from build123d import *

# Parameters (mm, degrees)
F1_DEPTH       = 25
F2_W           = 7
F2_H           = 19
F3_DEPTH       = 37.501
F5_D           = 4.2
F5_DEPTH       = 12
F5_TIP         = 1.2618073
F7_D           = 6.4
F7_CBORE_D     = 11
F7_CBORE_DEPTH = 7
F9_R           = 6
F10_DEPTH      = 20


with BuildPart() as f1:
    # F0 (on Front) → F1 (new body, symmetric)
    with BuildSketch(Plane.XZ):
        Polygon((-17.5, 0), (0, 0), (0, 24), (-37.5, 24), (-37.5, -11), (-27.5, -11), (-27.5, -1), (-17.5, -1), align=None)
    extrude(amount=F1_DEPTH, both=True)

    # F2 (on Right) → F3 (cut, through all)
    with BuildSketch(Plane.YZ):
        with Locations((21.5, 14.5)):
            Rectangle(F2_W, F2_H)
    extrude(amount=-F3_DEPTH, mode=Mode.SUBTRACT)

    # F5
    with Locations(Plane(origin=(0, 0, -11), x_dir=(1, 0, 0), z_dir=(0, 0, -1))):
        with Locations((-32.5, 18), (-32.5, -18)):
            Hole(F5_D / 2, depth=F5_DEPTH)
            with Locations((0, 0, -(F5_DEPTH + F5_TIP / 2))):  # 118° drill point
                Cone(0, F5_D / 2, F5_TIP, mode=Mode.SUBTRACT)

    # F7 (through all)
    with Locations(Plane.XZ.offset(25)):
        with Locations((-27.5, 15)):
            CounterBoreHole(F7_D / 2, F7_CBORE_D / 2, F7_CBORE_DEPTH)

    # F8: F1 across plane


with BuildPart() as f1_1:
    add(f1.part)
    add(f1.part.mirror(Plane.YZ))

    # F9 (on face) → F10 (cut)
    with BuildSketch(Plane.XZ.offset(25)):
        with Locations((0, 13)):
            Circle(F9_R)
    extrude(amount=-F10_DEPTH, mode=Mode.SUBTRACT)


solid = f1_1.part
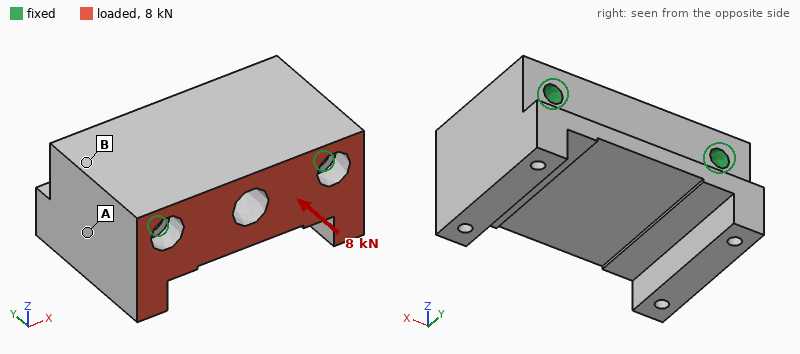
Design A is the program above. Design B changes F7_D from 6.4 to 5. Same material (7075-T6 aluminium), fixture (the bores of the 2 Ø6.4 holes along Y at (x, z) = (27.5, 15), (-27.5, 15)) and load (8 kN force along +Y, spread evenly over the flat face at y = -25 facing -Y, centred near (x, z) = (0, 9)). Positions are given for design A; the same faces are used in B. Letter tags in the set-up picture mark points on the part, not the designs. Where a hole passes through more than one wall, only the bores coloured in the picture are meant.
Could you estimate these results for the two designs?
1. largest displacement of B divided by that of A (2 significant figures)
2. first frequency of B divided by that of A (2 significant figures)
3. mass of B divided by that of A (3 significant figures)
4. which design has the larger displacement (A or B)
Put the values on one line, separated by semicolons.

1.1; 0.92; 1.01; B
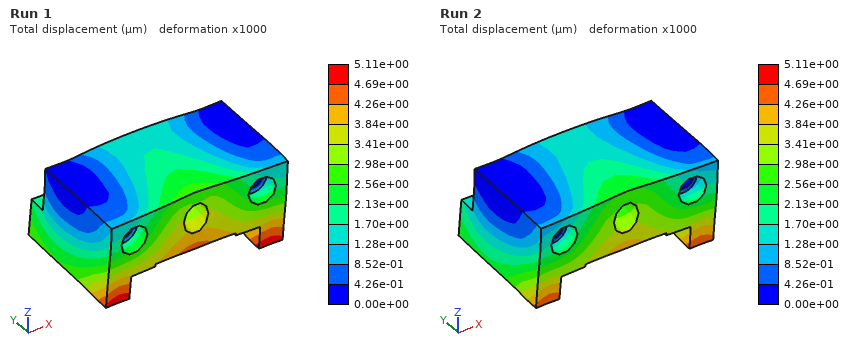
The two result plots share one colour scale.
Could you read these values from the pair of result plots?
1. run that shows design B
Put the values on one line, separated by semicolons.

Run 1
